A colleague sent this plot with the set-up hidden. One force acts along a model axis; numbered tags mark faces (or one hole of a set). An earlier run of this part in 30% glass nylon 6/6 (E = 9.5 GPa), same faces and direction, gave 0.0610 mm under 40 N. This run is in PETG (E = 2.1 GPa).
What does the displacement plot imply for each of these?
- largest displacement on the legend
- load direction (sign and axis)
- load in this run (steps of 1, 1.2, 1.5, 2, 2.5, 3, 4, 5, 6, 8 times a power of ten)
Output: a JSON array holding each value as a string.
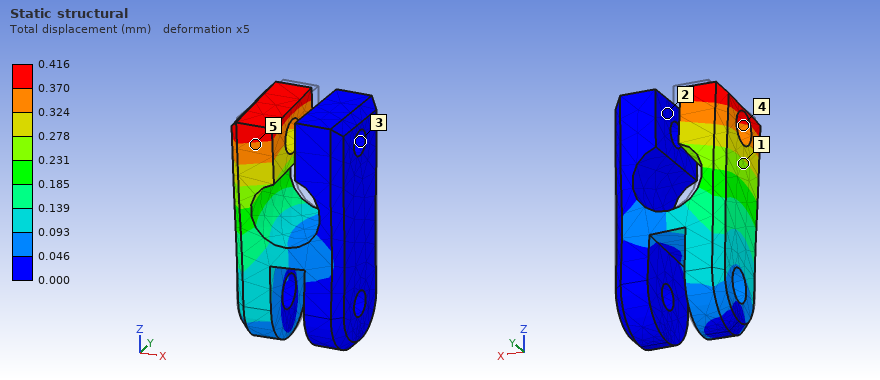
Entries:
["0.416 mm", "-Y", "60 N"]
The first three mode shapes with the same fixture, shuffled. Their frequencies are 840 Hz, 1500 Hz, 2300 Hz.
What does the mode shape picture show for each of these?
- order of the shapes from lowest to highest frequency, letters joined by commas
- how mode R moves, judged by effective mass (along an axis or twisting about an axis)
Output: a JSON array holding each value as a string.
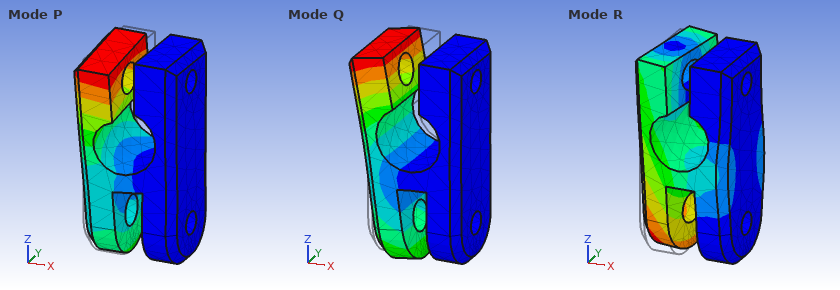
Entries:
["Q, P, R", "along Y"]
